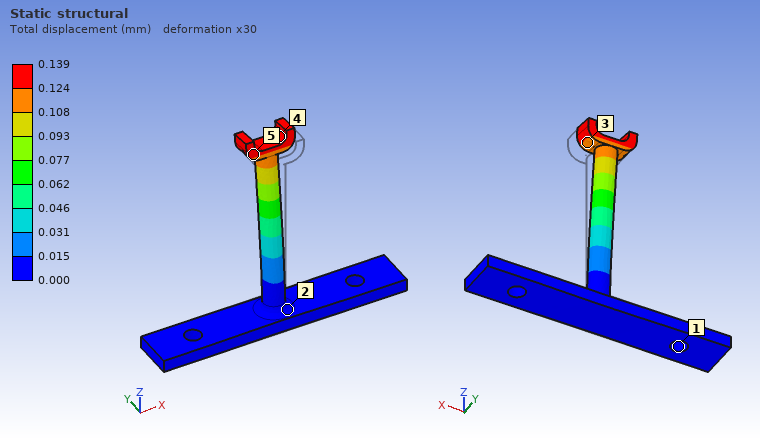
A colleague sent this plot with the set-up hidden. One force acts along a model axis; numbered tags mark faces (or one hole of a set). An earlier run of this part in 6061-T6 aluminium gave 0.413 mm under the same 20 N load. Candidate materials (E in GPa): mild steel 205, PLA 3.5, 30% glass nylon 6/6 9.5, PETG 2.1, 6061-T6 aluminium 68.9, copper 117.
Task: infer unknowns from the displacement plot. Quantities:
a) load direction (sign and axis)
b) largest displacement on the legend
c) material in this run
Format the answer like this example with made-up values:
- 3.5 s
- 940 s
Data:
- +Y
- 0.139 mm
- mild steel
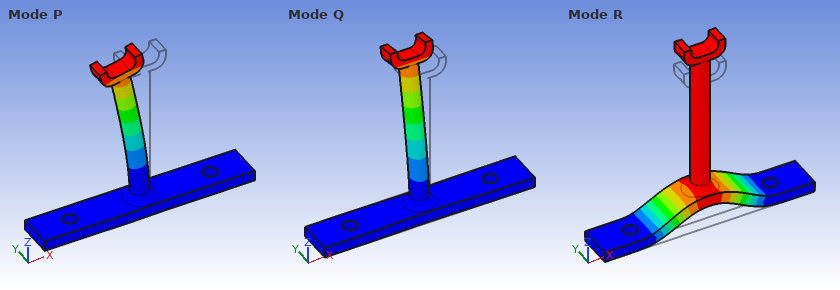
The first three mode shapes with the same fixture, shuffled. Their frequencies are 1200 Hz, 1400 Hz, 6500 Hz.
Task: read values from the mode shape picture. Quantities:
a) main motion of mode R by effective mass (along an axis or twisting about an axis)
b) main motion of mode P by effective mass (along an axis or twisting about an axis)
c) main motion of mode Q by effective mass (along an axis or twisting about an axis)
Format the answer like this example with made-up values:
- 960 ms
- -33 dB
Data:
- along Z
- along X
- along Y
